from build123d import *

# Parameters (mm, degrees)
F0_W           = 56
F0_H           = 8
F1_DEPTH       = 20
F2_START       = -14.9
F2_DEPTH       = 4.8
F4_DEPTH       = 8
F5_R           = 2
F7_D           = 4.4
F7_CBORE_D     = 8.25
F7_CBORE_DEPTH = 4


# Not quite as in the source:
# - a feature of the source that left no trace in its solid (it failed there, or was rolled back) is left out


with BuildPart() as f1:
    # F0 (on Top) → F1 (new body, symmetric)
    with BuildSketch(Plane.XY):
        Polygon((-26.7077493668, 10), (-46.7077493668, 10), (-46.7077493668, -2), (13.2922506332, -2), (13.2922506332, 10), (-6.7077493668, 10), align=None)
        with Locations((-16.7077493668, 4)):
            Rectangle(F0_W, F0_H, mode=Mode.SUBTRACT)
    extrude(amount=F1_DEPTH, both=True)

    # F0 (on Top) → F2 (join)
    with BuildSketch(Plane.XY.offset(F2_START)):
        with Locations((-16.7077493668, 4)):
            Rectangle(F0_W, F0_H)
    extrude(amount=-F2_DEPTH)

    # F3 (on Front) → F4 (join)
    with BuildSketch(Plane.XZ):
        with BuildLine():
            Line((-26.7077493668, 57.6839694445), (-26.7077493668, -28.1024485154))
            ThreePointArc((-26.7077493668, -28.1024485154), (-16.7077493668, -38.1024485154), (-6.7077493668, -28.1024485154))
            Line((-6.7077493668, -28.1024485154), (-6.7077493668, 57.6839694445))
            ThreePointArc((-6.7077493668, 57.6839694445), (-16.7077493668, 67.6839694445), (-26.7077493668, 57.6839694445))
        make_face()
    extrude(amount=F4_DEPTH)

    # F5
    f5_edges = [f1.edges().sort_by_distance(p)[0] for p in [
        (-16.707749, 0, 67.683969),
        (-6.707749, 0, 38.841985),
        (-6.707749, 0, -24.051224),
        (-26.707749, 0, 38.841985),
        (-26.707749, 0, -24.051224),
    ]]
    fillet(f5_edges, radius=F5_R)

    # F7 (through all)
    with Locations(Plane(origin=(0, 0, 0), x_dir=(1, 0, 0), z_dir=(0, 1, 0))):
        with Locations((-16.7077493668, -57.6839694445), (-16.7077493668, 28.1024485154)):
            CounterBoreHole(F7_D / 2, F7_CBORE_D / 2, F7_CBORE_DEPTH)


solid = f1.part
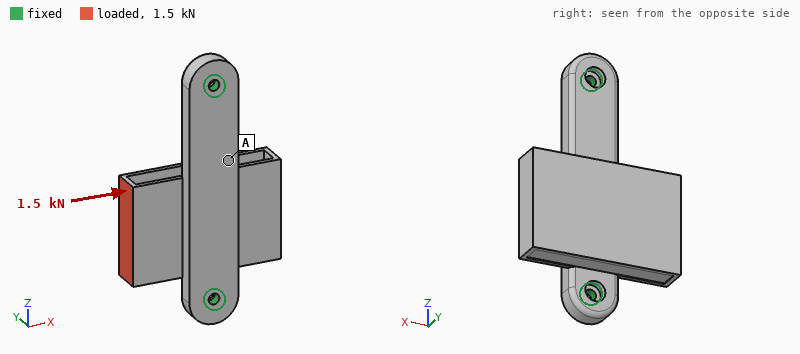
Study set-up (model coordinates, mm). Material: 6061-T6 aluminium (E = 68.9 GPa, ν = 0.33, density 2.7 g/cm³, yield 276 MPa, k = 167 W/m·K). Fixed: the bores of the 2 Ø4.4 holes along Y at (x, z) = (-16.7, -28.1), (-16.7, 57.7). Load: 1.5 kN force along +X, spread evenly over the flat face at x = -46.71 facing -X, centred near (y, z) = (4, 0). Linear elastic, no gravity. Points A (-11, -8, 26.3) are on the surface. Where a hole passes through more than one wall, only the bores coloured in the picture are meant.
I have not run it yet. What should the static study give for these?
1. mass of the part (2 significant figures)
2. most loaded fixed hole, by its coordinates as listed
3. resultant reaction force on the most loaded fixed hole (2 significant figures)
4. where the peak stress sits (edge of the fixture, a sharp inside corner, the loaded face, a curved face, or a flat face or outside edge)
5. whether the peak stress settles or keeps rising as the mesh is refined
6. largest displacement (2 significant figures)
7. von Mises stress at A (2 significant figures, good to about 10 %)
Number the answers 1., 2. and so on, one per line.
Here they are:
1. 73 g
2. (-16.7, -28.1)
3. 1.0 kN
4. edge of the fixture
5. keeps rising
6. 0.14 mm
7. 14 MPa
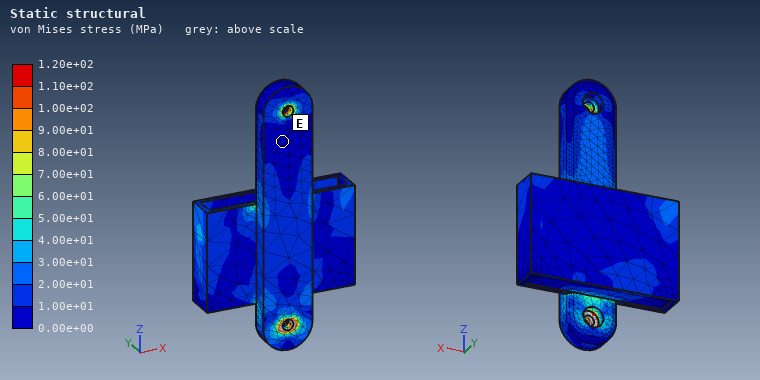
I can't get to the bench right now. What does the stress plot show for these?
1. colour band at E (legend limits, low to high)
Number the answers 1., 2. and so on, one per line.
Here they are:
1. 0.00e+00 to 1.00e+01 MPa
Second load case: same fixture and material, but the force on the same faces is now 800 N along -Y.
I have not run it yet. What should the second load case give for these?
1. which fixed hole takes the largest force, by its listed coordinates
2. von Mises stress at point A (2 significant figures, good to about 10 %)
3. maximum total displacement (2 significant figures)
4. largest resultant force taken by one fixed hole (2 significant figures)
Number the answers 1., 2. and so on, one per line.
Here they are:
1. (-16.7, -28.1)
2. 25 MPa
3. 0.47 mm
4. 850 N
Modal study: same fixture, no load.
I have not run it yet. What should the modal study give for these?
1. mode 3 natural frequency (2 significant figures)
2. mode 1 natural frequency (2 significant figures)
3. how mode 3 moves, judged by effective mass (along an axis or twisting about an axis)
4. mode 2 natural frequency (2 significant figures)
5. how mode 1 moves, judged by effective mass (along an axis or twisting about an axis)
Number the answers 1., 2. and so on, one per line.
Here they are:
1. 4300 Hz
2. 2100 Hz
3. along Y
4. 2300 Hz
5. along Y
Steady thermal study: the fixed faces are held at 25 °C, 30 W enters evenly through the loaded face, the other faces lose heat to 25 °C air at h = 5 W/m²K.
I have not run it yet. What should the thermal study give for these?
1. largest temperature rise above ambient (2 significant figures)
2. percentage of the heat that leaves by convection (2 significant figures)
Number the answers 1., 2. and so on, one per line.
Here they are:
1. 44 K
2. 4.4 %
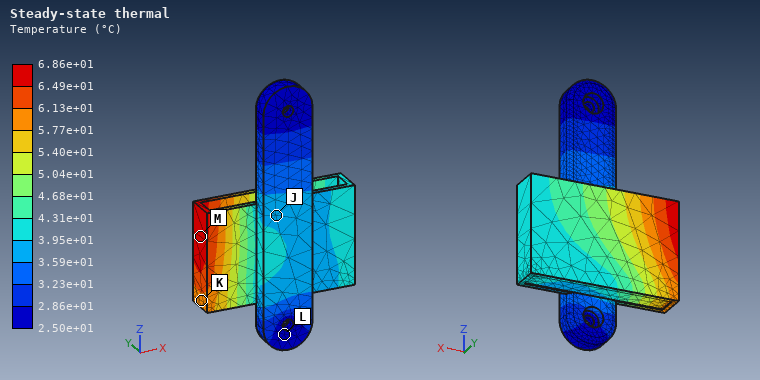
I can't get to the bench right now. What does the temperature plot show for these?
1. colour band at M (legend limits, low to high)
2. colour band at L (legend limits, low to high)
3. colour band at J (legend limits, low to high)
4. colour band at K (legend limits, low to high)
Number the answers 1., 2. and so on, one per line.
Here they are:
1. 6.49e+01 to 6.86e+01 °C
2. 2.50e+01 to 2.86e+01 °C
3. 3.59e+01 to 3.95e+01 °C
4. 5.77e+01 to 6.13e+01 °C
